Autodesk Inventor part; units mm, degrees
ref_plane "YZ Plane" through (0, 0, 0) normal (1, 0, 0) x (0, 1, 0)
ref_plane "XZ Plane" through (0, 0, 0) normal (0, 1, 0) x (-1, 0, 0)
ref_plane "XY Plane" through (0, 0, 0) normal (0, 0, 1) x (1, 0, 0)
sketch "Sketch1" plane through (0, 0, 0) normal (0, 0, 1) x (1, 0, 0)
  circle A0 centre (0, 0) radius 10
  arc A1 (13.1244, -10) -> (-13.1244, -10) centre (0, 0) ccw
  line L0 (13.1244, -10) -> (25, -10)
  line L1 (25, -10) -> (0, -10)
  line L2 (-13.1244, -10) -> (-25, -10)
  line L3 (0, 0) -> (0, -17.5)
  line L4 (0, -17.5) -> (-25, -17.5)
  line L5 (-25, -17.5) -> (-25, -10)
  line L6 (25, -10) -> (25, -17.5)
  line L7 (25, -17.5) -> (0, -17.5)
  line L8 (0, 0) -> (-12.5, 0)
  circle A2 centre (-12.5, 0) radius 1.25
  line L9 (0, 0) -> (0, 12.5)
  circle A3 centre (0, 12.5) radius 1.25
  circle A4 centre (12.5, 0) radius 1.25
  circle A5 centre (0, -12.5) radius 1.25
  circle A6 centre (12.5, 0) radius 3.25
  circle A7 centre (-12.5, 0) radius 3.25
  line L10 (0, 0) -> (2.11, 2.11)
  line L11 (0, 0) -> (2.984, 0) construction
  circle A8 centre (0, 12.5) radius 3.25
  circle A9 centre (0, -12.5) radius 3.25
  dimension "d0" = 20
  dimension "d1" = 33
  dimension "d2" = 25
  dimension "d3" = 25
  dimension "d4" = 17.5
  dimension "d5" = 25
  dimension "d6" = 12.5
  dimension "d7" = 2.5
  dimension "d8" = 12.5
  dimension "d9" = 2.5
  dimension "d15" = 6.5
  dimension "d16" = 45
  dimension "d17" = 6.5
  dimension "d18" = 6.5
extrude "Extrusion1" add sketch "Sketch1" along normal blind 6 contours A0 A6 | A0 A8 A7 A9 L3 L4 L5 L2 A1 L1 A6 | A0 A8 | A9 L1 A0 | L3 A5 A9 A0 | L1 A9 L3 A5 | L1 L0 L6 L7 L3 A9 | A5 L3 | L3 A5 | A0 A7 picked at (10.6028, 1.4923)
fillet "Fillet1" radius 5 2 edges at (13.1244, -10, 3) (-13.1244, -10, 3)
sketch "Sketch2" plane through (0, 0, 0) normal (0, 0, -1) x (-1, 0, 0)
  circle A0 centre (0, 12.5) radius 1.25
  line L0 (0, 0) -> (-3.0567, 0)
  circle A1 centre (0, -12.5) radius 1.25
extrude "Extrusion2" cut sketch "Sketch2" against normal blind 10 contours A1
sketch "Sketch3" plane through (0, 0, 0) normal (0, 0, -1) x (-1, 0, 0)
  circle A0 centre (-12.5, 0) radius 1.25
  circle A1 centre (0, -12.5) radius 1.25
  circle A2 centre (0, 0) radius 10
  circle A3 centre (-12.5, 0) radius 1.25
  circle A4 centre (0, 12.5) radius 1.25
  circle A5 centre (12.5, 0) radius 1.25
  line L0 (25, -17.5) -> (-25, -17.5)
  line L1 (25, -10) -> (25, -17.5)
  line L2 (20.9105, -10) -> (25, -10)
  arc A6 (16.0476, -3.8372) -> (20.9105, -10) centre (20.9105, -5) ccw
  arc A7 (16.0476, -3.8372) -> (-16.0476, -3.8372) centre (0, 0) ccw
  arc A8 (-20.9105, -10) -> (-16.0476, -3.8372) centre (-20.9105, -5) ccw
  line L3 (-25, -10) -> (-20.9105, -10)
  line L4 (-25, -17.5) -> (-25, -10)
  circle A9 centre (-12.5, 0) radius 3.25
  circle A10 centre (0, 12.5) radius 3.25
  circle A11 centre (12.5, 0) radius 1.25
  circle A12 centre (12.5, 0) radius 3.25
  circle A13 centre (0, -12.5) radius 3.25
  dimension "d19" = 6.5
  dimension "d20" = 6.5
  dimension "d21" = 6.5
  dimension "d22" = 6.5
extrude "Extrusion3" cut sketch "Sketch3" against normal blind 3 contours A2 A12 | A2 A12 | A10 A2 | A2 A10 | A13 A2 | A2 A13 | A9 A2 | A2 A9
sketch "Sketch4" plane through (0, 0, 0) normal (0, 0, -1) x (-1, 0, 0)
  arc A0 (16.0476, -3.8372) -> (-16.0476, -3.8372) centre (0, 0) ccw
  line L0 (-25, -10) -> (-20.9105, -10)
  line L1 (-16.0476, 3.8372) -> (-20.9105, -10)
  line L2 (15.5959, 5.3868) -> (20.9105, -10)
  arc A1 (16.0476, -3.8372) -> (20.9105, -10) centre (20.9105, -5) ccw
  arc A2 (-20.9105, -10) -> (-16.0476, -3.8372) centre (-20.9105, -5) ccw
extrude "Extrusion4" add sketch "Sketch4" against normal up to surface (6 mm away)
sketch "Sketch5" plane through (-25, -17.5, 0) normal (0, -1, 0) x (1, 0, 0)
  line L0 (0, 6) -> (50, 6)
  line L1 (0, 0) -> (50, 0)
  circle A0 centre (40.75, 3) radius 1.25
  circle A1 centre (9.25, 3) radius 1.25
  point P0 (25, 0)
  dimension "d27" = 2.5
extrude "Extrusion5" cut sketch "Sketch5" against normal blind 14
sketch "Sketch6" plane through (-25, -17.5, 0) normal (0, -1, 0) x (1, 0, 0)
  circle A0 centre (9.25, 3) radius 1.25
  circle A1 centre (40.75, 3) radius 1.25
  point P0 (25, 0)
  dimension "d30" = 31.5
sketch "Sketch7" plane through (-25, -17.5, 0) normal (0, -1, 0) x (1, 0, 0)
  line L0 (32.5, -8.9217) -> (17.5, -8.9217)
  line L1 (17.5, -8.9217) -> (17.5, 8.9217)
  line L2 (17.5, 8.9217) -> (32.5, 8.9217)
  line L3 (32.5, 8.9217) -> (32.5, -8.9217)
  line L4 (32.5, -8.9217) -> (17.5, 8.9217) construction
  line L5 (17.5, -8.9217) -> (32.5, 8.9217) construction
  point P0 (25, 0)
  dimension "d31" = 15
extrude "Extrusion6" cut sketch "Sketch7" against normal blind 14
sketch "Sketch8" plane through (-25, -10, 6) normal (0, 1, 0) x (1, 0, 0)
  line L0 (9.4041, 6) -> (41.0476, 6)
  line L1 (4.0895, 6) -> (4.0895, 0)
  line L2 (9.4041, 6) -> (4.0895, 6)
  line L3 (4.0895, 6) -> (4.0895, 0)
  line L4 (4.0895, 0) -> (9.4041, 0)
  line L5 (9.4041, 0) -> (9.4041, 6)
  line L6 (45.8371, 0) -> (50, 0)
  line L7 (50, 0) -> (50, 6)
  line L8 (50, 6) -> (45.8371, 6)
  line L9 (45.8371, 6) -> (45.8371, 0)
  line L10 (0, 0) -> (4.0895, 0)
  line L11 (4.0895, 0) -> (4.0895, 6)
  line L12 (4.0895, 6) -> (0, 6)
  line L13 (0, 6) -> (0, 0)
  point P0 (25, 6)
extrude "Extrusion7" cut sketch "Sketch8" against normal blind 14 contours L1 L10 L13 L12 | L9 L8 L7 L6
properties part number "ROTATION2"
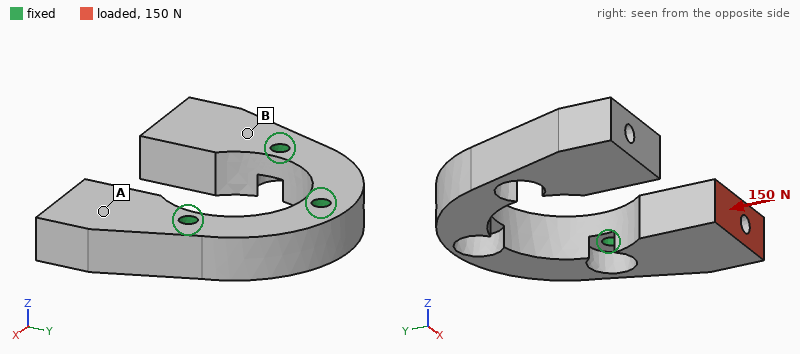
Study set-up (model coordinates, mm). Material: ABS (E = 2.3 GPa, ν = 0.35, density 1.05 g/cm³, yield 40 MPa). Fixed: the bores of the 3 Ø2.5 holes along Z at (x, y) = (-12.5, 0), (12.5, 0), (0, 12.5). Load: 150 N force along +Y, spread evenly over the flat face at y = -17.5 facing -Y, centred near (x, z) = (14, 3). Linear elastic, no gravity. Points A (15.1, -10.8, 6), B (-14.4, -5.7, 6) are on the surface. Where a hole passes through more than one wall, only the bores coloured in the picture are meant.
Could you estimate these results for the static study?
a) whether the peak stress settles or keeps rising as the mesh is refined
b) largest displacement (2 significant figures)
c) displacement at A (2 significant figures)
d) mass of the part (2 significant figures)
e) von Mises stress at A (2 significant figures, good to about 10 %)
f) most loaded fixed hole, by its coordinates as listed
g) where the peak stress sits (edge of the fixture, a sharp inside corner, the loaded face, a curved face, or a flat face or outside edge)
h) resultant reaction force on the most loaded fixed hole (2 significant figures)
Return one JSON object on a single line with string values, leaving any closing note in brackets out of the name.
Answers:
{"whether the peak stress settles or keeps rising as the mesh is refined": "keeps rising", "largest displacement": "0.16 mm", "displacement at A": "0.082 mm", "mass of the part": "3.8 g", "von Mises stress at A": "2.4 MPa", "most loaded fixed hole, by its coordinates as listed": "(12.5, 0)", "where the peak stress sits": "edge of the fixture", "resultant reaction force on the most loaded fixed hole": "140 N"}
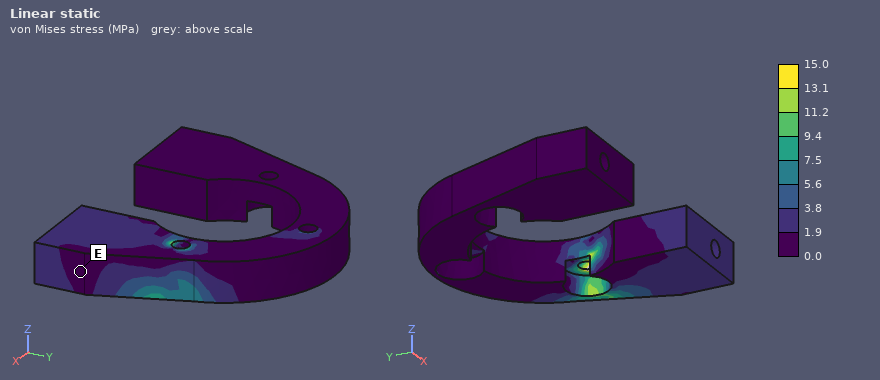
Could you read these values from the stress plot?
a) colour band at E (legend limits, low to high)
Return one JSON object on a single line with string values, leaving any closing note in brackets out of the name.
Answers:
{"colour band at E": "0.0 to 1.9 MPa"}
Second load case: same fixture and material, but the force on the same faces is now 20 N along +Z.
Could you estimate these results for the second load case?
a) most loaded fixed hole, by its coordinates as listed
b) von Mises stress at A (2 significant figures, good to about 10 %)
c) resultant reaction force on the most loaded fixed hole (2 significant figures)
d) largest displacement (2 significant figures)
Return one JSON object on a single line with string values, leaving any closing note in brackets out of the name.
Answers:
{"most loaded fixed hole, by its coordinates as listed": "(12.5, 0)", "von Mises stress at A": "2.0 MPa", "resultant reaction force on the most loaded fixed hole": "25 N", "largest displacement": "0.31 mm"}
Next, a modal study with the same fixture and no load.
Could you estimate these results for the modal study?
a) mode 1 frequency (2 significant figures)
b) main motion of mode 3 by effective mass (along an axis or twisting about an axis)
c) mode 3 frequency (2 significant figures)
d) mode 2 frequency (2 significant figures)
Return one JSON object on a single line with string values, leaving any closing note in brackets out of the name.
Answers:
{"mode 1 frequency": "2000 Hz", "main motion of mode 3 by effective mass": "along X", "mode 3 frequency": "2800 Hz", "mode 2 frequency": "2000 Hz"}
